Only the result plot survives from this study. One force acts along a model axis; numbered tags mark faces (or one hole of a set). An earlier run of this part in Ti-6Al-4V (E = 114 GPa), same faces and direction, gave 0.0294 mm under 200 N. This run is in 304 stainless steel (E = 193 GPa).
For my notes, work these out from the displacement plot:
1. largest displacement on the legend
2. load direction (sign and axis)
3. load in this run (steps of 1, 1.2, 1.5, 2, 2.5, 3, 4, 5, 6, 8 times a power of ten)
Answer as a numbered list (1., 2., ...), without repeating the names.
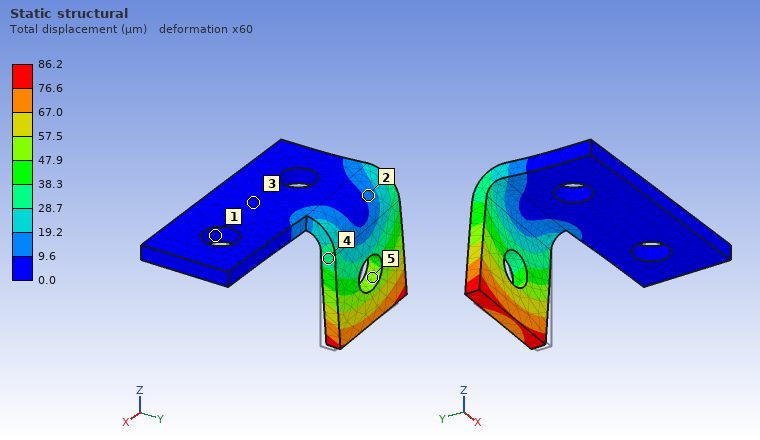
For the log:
1. 86.2 µm
2. -X
3. 1 kN
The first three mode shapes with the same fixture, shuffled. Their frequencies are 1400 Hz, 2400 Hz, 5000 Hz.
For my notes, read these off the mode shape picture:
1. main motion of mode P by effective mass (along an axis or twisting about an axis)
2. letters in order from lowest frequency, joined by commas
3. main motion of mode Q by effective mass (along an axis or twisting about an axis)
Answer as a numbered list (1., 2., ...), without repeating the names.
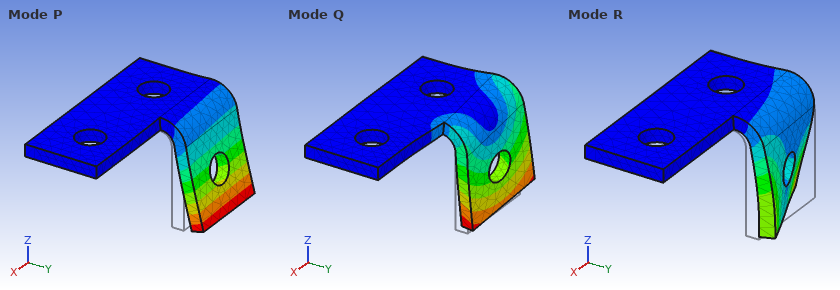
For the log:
1. along Y
2. P, Q, R
3. along X
